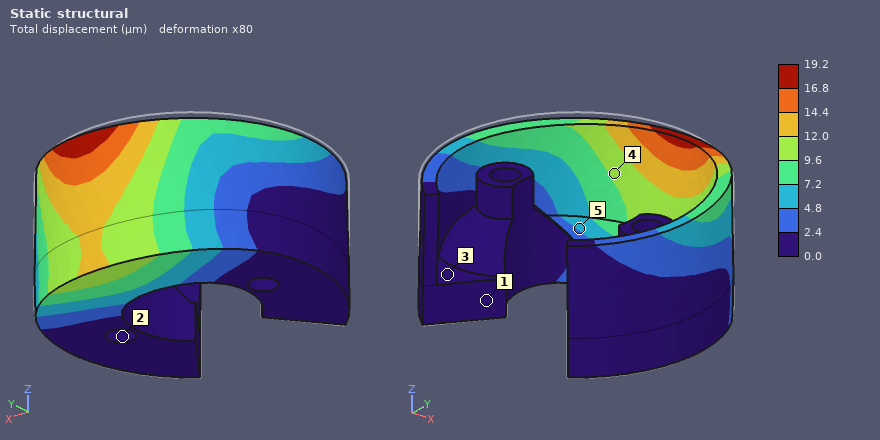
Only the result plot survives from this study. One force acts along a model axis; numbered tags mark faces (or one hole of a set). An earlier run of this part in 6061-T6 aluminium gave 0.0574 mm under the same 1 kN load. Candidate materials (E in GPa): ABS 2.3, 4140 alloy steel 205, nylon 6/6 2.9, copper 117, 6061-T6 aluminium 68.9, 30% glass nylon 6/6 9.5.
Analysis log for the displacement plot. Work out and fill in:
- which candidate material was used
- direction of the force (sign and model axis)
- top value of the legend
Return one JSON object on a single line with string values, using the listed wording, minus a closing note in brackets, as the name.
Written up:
{"which candidate material was used": "4140 alloy steel", "direction of the force": "-Z", "top value of the legend": "19.2 µm"}
